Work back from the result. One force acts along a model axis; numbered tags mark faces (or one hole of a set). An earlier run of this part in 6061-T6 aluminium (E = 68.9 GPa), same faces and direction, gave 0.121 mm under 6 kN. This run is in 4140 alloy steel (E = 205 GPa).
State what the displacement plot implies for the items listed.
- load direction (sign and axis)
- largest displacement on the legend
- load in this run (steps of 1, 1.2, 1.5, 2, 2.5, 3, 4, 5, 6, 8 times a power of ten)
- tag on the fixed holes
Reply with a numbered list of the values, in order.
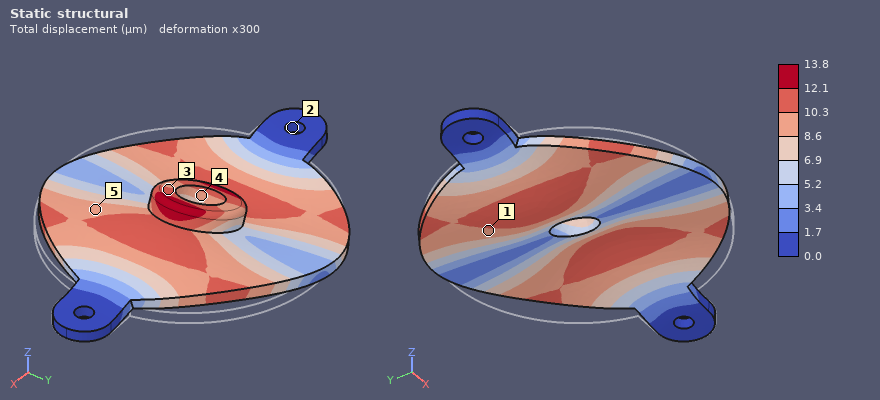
1. -X
2. 13.8 µm
3. 2 kN
4. 2
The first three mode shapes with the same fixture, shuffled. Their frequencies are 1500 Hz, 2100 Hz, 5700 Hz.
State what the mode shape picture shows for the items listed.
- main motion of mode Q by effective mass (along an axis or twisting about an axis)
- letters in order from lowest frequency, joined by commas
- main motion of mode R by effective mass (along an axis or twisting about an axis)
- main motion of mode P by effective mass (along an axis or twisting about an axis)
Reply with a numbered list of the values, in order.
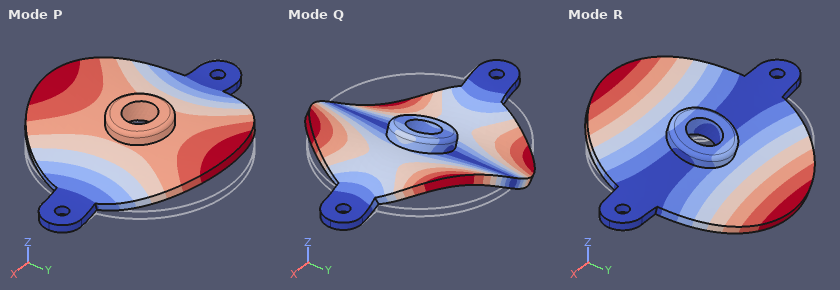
1. twisting about Y
2. R, P, Q
3. twisting about X
4. along Z
